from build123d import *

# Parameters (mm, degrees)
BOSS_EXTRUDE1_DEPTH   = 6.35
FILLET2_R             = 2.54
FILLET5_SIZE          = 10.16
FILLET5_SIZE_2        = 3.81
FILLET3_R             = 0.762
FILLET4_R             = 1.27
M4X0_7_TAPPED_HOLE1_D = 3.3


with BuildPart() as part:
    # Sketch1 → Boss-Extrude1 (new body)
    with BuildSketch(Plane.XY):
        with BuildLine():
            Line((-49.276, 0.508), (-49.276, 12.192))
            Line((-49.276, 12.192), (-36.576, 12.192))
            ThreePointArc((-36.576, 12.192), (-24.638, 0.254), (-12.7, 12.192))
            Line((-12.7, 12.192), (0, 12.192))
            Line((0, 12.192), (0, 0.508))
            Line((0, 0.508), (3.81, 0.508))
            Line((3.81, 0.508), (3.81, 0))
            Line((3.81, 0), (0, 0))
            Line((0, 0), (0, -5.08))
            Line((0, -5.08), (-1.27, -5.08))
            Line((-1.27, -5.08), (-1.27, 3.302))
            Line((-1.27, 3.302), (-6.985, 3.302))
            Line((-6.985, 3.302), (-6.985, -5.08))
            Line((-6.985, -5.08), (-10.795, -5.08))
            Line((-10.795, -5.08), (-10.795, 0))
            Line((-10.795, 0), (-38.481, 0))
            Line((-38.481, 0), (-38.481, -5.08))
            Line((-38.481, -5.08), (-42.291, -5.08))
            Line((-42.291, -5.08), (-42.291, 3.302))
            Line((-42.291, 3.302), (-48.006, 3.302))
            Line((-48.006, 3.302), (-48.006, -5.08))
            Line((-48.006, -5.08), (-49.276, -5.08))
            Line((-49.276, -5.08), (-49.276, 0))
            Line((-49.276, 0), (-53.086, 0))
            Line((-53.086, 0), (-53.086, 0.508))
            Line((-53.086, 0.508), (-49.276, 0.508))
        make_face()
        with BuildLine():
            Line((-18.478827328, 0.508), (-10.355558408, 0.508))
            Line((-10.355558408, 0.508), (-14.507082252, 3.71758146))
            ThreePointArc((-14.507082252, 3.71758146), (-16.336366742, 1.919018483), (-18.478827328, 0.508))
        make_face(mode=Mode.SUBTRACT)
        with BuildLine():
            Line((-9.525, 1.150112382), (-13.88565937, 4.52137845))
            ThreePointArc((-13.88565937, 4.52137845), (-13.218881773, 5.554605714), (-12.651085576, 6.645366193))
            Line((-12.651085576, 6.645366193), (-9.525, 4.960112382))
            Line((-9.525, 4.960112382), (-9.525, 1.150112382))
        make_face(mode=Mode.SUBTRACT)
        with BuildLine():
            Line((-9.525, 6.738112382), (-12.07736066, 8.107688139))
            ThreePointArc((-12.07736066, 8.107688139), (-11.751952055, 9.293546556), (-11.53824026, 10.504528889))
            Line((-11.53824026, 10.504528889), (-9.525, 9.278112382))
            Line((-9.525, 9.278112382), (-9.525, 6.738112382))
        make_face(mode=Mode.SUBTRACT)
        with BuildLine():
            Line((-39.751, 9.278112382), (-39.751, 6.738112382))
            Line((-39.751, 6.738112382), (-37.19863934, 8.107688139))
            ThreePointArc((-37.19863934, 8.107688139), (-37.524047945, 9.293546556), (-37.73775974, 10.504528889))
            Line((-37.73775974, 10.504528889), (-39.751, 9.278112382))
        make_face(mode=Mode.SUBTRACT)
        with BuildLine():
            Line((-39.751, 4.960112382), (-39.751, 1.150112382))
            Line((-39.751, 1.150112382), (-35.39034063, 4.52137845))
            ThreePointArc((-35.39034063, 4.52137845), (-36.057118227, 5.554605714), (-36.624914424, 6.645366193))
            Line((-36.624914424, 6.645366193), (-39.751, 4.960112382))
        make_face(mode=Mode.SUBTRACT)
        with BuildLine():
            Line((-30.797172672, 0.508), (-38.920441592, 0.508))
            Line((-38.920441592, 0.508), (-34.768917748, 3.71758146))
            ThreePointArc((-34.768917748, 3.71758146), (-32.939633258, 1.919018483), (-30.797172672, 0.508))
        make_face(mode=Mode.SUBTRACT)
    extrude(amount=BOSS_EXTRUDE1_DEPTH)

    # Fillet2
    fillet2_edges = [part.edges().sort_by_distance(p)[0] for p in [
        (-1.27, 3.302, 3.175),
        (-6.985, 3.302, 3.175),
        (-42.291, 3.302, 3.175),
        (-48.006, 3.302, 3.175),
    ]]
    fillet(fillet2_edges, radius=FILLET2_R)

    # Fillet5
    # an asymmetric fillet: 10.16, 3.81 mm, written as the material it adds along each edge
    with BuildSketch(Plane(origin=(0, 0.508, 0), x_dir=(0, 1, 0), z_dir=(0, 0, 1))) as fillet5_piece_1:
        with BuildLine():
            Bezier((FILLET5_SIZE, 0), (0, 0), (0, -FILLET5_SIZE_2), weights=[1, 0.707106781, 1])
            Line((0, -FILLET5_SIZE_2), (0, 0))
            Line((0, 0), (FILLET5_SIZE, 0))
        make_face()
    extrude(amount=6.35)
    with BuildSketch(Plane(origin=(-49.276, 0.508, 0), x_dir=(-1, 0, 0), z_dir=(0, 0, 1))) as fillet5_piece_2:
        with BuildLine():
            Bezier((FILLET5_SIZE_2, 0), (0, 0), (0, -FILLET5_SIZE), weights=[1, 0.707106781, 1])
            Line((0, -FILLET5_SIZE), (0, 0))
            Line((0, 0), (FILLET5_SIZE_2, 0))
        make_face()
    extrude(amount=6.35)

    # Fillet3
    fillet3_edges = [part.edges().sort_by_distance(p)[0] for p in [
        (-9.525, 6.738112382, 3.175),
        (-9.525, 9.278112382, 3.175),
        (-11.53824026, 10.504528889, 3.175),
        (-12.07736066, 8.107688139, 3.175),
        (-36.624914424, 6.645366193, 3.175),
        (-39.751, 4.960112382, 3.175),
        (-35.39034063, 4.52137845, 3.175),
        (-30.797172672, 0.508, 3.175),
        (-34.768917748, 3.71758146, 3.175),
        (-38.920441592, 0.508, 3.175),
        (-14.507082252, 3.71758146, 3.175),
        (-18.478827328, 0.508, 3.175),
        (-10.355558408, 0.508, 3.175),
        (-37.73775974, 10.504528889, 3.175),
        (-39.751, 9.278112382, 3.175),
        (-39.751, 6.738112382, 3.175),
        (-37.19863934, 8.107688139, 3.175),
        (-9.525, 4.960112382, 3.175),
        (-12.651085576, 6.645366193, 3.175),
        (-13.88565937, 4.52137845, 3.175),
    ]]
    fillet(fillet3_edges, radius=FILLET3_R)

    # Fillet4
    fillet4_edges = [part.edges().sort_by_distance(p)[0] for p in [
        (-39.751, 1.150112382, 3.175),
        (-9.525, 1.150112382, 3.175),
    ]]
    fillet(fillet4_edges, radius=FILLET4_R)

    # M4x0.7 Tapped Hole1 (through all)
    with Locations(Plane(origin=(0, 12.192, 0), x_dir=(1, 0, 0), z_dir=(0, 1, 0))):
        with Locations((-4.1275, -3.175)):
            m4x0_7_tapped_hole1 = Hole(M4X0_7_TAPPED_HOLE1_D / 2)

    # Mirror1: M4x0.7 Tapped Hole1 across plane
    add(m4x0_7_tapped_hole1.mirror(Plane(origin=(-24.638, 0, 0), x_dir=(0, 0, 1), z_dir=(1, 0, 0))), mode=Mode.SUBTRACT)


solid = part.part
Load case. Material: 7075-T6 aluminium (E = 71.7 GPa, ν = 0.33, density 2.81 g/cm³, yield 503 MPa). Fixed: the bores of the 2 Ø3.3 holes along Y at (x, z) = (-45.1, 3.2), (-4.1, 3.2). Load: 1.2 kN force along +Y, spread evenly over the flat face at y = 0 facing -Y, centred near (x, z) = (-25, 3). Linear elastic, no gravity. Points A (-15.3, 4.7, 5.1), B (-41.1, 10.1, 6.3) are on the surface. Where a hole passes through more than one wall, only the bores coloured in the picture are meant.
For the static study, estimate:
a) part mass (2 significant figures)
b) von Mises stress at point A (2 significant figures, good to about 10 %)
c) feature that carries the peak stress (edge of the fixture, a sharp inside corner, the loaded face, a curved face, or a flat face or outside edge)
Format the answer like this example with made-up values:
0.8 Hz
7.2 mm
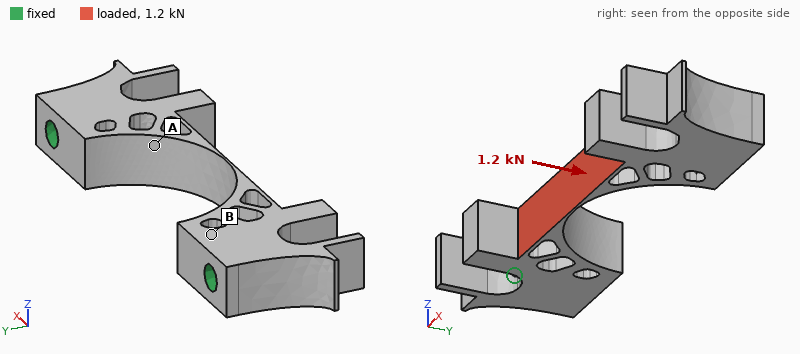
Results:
6.1 g
110 MPa
the loaded face
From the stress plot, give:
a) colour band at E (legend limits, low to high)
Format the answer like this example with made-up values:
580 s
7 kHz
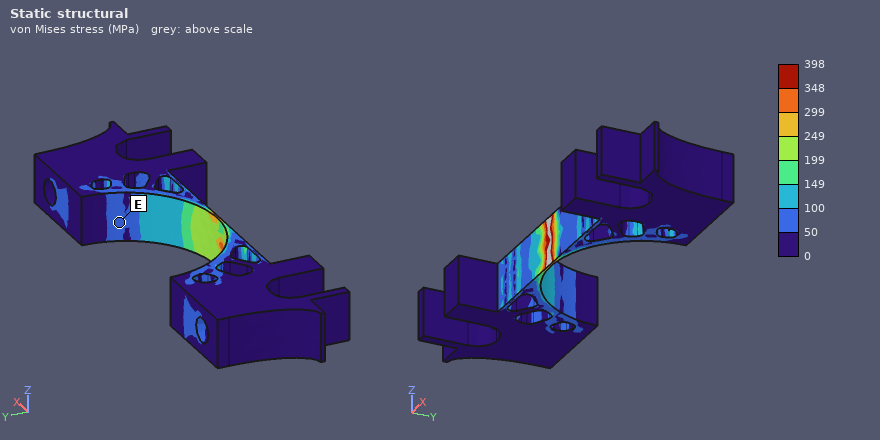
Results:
50 to 100 MPa
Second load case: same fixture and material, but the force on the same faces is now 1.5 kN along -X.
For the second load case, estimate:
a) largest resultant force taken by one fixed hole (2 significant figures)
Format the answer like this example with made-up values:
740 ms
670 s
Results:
750 N
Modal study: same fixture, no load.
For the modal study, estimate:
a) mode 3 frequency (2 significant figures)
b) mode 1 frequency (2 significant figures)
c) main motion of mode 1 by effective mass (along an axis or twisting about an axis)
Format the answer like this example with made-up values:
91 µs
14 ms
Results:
26 kHz
21 kHz
along Z
